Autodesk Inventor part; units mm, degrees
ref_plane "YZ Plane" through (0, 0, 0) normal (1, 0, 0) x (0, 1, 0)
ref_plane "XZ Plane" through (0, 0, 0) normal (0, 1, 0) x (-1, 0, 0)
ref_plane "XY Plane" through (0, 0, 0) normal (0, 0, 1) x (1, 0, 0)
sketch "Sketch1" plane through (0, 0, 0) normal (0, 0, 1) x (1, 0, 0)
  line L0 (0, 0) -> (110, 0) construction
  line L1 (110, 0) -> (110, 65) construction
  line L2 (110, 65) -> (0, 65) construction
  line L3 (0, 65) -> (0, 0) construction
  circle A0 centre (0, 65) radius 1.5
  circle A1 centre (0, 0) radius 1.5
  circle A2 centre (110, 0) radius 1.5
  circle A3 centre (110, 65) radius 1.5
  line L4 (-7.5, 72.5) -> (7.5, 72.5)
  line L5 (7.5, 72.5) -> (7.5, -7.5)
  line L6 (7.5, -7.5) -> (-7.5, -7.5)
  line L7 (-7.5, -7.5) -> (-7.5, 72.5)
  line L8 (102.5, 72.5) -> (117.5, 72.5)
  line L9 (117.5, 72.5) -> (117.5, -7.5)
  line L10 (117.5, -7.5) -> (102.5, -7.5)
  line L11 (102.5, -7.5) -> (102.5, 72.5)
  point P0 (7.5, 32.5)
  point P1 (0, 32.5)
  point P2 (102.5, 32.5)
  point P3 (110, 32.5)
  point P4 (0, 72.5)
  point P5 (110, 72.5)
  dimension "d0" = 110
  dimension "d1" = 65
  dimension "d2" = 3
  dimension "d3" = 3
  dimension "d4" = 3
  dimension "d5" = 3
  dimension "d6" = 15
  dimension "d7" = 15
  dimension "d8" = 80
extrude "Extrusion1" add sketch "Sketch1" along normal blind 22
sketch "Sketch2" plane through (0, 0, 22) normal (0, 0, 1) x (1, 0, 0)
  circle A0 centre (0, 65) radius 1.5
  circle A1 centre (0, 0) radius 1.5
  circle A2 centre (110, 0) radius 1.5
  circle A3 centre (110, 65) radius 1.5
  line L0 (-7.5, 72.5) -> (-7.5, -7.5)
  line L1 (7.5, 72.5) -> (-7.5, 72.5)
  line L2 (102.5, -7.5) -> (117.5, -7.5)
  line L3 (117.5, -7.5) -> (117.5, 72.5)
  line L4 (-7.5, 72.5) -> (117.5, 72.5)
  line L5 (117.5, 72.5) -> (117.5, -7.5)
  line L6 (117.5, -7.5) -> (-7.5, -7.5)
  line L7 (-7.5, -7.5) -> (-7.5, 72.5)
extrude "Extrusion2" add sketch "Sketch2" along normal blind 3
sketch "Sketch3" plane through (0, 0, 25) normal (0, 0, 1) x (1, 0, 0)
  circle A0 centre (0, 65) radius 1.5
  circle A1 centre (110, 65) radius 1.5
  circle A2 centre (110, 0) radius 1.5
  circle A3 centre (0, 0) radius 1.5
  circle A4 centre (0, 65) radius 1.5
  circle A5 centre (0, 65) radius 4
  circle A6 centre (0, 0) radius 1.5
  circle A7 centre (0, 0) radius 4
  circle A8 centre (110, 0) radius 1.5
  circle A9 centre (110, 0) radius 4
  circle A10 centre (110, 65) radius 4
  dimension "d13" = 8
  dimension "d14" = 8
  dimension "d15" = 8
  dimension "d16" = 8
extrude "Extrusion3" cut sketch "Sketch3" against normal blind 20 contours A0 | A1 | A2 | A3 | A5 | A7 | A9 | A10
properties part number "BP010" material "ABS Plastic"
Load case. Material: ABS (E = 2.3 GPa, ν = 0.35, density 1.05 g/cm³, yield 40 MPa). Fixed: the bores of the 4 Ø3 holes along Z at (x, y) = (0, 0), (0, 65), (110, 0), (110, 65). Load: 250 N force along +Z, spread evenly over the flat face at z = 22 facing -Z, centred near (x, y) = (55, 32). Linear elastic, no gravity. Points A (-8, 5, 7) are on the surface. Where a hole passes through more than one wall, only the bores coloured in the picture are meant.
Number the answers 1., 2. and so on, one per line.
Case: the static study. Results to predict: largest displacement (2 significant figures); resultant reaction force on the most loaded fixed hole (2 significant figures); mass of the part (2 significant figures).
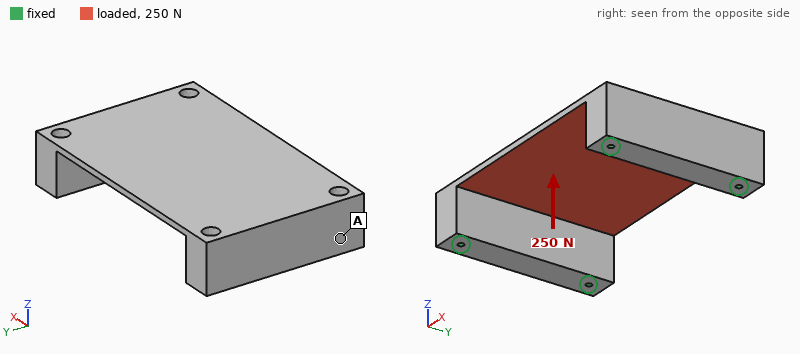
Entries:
1. 1.6 mm
2. 94 N
3. 83 g
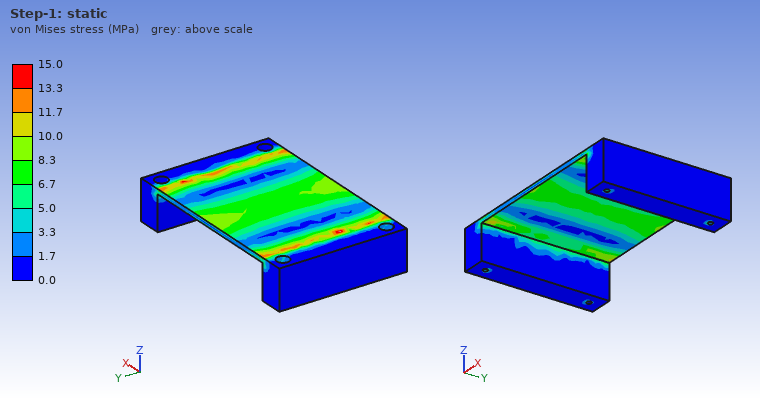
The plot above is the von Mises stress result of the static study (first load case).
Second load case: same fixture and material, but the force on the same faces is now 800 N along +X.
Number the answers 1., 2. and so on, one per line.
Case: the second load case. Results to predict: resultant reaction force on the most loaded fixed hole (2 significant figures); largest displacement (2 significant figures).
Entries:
1. 200 N
2. 0.74 mm
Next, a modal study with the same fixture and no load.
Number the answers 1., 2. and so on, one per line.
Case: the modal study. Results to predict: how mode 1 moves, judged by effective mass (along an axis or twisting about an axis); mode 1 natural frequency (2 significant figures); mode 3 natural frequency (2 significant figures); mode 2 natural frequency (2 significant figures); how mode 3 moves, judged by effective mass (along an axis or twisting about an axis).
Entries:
1. along Z
2. 490 Hz
3. 790 Hz
4. 610 Hz
5. along X
